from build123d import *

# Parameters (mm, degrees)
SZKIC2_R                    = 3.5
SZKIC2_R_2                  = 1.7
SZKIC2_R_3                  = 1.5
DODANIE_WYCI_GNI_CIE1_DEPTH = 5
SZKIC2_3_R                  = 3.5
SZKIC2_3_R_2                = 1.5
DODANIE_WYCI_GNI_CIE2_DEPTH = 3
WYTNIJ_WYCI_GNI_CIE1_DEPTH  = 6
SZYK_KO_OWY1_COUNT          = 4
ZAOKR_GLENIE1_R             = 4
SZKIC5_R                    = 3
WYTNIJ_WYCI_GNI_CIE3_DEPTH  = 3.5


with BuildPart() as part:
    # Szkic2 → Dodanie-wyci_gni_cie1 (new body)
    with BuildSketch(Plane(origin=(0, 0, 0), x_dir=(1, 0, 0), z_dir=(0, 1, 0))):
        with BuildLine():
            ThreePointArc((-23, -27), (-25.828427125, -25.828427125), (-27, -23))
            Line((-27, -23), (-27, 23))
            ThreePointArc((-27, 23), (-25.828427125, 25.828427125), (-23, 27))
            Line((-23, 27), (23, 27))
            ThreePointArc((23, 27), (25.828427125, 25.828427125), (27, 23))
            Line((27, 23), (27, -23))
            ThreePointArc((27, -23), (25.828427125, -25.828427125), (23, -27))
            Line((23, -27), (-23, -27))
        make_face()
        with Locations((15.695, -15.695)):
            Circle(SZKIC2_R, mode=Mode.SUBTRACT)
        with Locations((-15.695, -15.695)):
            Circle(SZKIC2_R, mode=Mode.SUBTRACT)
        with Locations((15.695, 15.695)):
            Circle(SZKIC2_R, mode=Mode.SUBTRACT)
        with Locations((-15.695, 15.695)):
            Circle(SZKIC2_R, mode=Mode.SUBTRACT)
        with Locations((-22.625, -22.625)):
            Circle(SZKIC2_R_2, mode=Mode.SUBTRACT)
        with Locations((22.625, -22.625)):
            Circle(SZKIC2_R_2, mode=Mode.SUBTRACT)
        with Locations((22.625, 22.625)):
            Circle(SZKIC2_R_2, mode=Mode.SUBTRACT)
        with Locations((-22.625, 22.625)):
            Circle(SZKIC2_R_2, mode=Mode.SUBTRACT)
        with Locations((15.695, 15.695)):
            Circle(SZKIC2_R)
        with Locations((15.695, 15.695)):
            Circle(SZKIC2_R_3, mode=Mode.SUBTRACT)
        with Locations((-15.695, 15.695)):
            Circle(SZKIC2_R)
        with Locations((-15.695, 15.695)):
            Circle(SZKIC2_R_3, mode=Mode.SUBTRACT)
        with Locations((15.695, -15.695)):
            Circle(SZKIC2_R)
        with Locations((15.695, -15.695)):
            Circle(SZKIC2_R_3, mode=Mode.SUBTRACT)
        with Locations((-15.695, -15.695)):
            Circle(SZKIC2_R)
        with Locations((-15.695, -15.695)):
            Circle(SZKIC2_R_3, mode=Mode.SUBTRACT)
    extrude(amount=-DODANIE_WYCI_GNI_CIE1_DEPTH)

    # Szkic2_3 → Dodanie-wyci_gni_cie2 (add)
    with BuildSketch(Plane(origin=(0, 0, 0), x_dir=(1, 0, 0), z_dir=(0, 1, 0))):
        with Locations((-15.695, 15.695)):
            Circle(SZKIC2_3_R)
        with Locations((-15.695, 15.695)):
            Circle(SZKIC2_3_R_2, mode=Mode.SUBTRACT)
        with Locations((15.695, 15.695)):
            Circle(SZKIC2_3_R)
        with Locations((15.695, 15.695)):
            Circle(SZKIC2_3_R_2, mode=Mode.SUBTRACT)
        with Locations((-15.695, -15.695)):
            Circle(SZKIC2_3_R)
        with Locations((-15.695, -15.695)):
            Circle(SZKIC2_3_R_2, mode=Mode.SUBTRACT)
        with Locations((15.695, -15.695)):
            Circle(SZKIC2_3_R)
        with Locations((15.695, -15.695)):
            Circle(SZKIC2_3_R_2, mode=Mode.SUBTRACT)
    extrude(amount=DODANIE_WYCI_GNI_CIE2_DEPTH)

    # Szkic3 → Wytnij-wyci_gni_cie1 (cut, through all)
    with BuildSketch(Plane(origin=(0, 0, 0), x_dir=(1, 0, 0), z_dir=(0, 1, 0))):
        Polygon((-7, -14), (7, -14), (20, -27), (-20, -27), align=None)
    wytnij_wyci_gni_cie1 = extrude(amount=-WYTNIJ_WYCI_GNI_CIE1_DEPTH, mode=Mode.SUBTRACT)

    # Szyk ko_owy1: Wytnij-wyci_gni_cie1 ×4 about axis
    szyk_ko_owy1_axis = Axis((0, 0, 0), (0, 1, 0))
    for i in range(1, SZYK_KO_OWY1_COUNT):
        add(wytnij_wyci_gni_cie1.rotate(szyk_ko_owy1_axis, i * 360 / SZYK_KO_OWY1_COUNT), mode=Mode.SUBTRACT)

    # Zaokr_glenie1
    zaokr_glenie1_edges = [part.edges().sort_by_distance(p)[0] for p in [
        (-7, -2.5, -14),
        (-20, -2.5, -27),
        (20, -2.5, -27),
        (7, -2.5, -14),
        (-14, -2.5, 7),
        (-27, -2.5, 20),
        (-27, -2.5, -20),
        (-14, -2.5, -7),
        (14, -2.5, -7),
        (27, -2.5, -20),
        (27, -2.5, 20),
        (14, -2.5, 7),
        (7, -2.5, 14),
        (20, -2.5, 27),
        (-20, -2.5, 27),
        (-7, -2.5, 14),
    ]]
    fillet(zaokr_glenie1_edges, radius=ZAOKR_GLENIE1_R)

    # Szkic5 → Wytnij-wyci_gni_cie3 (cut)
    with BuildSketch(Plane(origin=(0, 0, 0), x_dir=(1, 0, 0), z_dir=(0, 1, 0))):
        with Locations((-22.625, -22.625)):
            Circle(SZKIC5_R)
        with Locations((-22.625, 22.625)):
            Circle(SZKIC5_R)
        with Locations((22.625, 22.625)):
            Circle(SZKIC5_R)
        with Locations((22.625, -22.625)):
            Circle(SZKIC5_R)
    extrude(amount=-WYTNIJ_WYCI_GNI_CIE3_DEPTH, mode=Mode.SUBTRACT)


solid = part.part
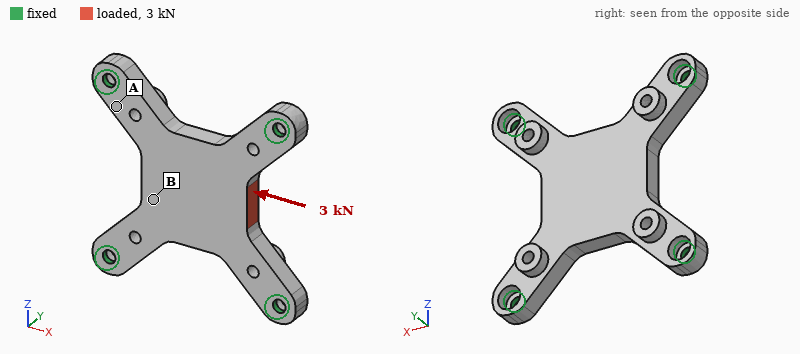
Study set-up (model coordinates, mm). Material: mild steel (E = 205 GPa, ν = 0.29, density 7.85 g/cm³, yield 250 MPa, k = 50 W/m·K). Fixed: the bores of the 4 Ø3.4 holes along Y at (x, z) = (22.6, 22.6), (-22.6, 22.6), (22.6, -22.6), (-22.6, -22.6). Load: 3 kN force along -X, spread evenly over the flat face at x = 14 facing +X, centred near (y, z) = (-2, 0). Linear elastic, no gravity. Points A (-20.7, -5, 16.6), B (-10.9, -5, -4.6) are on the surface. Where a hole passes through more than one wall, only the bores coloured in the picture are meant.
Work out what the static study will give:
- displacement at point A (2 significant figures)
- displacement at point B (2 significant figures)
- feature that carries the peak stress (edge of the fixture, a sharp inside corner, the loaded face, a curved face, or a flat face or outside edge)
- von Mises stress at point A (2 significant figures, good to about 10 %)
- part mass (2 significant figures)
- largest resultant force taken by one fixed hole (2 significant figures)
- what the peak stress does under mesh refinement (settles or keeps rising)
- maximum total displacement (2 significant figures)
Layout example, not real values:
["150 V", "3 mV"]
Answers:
["2.7 µm", "6.1 µm", "edge of the fixture", "41 MPa", "57 g", "980 N", "keeps rising", "9.8 µm"]
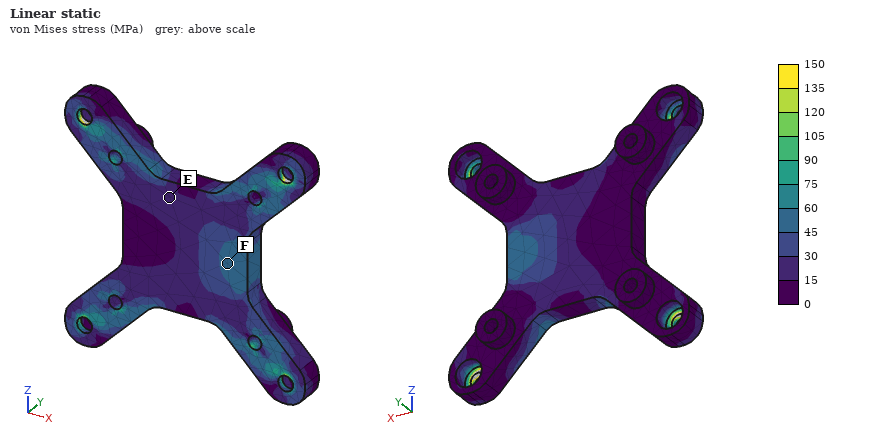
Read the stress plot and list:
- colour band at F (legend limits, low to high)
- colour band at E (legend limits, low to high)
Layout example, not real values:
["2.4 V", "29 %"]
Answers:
["45 to 60 MPa", "15 to 30 MPa"]
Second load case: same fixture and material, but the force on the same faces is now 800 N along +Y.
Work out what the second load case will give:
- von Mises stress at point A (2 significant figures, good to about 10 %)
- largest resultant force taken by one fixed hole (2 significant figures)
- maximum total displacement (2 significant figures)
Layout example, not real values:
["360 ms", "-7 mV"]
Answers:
["26 MPa", "550 N", "34 µm"]
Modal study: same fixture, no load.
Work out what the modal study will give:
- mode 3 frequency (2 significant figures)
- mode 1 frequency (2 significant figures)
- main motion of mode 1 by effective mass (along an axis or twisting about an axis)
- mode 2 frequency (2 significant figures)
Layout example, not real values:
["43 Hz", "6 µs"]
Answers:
["12 kHz", "5600 Hz", "along Y", "12 kHz"]
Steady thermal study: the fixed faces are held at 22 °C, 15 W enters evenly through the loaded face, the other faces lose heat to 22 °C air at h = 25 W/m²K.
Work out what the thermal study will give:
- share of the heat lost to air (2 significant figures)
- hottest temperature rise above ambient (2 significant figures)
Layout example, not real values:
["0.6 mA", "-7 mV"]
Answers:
["16 %", "66 K"]
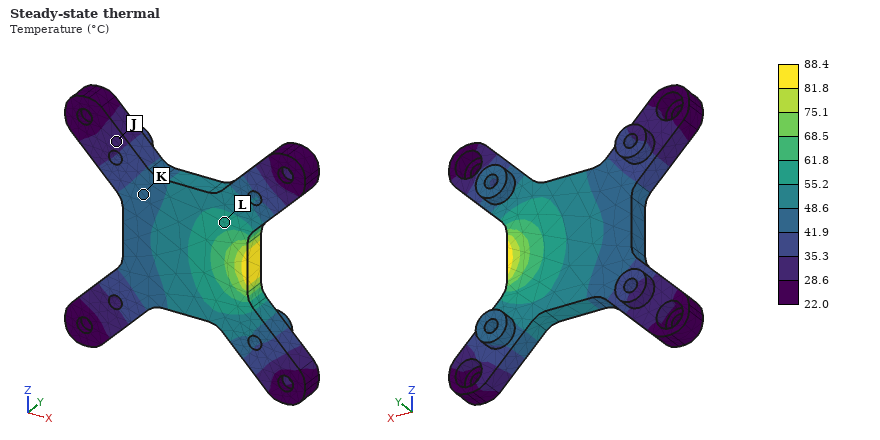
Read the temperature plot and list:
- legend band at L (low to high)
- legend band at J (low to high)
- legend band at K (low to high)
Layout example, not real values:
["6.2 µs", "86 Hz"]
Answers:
["55.2 to 61.8 °C", "28.6 to 35.3 °C", "41.9 to 48.6 °C"]
